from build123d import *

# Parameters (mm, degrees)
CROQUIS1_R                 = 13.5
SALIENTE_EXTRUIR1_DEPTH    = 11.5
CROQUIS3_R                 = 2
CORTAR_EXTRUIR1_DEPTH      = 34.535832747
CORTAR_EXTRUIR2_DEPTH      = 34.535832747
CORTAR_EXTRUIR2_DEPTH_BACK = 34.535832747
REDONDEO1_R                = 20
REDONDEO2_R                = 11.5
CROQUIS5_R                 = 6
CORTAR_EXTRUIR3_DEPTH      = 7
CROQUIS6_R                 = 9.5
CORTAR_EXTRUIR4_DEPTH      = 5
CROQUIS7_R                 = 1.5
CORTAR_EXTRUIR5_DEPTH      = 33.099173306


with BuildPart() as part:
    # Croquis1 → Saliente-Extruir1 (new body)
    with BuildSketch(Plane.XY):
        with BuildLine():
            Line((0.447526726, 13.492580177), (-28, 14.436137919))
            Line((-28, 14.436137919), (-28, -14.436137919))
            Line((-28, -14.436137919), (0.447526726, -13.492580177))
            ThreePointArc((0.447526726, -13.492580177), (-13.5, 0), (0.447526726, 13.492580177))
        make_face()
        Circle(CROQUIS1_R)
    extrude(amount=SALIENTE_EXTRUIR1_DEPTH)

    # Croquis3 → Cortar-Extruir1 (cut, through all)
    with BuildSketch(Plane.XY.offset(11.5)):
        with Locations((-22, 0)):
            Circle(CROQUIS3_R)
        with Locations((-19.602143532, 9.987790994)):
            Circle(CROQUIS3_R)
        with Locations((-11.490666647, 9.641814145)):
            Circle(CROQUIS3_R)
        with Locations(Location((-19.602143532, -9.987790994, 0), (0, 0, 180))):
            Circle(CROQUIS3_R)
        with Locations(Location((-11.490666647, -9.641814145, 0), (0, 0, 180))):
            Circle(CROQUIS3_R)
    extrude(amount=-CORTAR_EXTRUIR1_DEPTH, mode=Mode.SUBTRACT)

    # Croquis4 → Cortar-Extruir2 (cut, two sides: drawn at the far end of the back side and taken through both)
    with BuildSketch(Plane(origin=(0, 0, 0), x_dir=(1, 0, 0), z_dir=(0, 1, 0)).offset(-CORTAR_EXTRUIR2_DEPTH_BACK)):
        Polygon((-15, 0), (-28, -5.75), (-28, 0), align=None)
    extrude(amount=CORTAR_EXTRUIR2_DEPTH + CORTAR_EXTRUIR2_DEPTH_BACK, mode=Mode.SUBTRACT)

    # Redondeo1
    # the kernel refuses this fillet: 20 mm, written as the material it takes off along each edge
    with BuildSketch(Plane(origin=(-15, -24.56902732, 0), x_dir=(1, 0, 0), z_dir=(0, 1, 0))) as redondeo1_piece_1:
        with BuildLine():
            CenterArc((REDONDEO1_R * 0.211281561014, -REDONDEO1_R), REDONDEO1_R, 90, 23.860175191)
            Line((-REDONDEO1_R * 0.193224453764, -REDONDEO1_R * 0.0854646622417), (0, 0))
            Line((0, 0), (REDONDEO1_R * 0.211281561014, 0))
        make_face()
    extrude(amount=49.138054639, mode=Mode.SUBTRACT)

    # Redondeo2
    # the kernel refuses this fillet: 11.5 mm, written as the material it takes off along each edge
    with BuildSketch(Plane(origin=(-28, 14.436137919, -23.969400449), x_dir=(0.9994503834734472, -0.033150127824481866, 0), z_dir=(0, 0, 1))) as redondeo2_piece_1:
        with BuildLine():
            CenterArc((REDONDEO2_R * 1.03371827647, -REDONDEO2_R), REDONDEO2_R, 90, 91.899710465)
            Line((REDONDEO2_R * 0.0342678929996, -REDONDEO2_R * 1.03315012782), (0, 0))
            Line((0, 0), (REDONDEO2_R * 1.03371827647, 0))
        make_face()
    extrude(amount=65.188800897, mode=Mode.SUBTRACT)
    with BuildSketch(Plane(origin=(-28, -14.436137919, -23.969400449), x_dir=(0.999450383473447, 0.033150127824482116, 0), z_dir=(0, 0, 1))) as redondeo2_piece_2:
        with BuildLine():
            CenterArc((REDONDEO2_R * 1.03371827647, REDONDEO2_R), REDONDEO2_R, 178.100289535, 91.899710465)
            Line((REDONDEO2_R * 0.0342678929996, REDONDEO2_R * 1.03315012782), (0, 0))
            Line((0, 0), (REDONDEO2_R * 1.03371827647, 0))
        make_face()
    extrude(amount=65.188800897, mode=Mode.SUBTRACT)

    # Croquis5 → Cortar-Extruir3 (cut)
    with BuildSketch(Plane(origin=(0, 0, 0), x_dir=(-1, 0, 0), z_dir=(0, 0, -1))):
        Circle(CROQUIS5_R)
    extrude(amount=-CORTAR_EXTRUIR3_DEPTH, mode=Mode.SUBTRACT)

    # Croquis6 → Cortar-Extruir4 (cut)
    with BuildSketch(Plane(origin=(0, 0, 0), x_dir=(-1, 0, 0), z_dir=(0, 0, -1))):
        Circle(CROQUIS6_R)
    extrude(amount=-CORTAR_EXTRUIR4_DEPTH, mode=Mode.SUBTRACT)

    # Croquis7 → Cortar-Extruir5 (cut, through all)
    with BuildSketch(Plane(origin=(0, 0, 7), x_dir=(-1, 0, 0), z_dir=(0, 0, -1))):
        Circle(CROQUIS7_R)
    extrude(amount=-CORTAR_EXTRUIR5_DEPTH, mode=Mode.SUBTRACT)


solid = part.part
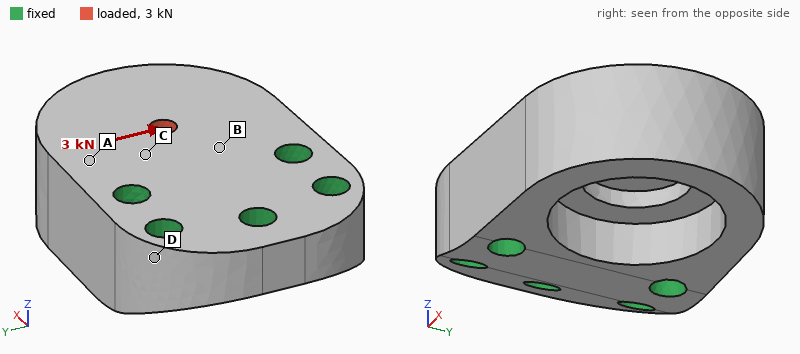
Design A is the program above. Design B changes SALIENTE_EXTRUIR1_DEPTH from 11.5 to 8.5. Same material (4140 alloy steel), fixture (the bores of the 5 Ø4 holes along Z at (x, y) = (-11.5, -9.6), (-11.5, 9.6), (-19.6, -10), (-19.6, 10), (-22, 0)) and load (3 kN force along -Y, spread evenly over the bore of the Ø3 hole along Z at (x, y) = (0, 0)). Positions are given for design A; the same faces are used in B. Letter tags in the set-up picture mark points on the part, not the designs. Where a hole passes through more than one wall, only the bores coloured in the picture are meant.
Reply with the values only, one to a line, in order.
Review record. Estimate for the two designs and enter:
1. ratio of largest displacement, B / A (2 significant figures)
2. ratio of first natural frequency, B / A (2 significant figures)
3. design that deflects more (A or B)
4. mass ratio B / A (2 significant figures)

2.3
0.79
B
0.67
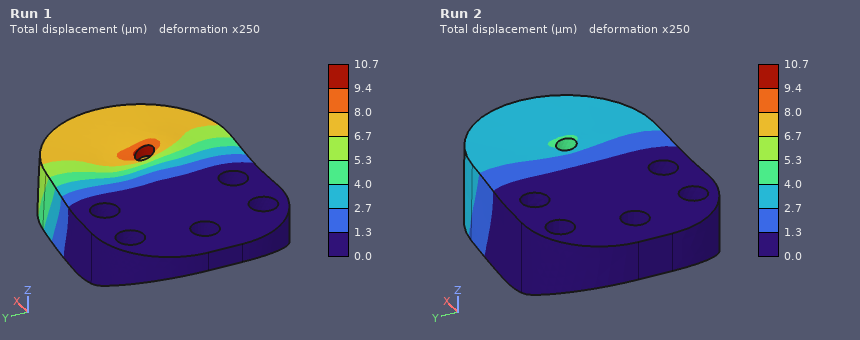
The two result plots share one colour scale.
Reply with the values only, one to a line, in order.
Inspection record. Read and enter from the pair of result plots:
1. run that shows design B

Run 1
